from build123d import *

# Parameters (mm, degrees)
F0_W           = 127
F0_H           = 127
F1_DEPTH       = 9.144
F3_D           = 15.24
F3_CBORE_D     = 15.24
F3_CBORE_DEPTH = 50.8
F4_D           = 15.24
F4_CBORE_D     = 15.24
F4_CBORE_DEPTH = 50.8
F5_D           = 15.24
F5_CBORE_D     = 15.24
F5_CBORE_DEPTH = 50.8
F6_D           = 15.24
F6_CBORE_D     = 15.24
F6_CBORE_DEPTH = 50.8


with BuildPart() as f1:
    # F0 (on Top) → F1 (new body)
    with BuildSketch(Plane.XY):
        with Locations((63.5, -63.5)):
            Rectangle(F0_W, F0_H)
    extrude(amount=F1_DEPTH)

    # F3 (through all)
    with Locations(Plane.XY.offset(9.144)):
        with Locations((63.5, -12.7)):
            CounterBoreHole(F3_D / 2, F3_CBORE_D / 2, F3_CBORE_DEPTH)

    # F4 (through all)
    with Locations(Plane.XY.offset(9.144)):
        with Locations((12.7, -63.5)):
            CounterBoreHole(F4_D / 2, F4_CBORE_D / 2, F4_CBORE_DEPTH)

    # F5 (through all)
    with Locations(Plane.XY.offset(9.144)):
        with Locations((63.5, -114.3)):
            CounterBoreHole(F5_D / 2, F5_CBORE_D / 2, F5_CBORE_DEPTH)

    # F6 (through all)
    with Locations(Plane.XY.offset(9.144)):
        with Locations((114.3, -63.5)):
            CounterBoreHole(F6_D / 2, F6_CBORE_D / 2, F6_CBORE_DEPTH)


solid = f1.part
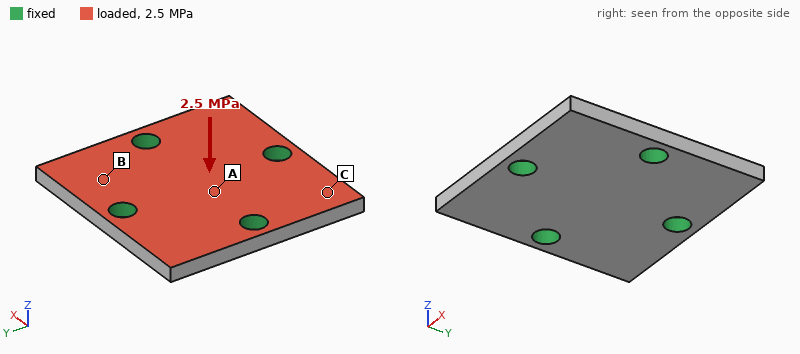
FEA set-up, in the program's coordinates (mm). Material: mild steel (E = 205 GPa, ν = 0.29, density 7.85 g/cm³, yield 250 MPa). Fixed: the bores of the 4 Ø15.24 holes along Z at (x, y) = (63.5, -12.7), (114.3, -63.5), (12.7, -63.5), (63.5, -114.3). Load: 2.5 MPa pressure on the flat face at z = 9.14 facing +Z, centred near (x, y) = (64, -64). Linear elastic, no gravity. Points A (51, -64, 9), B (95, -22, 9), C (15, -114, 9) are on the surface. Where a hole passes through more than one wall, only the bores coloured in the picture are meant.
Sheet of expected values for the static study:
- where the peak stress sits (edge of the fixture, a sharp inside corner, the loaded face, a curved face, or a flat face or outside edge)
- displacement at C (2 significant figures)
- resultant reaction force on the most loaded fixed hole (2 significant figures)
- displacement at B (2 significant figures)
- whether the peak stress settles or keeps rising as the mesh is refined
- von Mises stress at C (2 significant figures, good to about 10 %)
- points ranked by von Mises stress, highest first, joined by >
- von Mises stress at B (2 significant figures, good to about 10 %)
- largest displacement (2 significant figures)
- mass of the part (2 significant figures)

edge of the fixture
54 µm
9.6 kN
25 µm
keeps rising
43 MPa
B > C > A
57 MPa
93 µm
1.1 kg
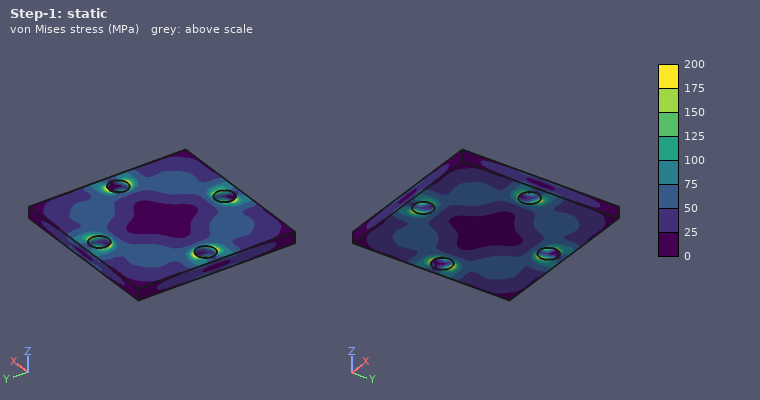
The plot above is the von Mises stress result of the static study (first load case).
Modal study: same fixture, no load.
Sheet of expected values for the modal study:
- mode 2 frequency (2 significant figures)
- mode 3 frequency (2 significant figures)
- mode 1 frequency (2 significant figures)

4300 Hz
4300 Hz
4200 Hz
